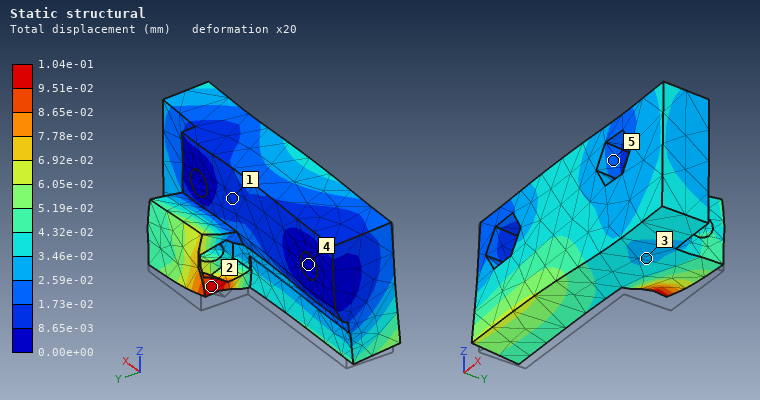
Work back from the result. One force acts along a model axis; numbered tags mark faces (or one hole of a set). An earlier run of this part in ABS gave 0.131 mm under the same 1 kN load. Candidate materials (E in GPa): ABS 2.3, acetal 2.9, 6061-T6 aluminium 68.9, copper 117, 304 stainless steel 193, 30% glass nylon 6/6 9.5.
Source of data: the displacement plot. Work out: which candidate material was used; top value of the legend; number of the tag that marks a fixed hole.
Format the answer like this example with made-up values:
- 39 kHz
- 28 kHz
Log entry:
- acetal
- 1.04e-01 mm
- 4
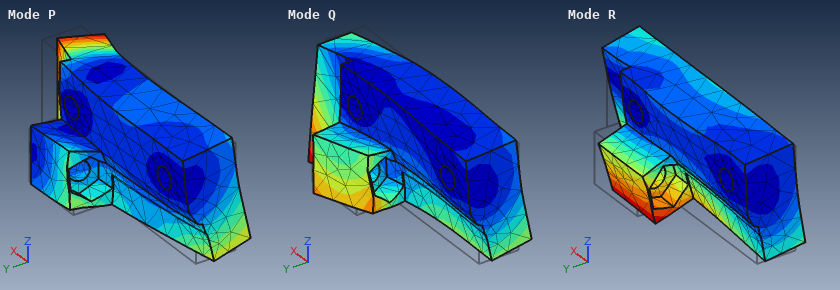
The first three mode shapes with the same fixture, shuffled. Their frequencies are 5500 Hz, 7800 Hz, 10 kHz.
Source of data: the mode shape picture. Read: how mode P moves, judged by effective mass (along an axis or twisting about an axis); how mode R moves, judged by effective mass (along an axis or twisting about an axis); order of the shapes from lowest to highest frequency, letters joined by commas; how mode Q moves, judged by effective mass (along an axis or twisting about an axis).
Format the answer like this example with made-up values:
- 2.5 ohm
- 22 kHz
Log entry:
- along X
- along Y
- R, Q, P
- twisting about Z
